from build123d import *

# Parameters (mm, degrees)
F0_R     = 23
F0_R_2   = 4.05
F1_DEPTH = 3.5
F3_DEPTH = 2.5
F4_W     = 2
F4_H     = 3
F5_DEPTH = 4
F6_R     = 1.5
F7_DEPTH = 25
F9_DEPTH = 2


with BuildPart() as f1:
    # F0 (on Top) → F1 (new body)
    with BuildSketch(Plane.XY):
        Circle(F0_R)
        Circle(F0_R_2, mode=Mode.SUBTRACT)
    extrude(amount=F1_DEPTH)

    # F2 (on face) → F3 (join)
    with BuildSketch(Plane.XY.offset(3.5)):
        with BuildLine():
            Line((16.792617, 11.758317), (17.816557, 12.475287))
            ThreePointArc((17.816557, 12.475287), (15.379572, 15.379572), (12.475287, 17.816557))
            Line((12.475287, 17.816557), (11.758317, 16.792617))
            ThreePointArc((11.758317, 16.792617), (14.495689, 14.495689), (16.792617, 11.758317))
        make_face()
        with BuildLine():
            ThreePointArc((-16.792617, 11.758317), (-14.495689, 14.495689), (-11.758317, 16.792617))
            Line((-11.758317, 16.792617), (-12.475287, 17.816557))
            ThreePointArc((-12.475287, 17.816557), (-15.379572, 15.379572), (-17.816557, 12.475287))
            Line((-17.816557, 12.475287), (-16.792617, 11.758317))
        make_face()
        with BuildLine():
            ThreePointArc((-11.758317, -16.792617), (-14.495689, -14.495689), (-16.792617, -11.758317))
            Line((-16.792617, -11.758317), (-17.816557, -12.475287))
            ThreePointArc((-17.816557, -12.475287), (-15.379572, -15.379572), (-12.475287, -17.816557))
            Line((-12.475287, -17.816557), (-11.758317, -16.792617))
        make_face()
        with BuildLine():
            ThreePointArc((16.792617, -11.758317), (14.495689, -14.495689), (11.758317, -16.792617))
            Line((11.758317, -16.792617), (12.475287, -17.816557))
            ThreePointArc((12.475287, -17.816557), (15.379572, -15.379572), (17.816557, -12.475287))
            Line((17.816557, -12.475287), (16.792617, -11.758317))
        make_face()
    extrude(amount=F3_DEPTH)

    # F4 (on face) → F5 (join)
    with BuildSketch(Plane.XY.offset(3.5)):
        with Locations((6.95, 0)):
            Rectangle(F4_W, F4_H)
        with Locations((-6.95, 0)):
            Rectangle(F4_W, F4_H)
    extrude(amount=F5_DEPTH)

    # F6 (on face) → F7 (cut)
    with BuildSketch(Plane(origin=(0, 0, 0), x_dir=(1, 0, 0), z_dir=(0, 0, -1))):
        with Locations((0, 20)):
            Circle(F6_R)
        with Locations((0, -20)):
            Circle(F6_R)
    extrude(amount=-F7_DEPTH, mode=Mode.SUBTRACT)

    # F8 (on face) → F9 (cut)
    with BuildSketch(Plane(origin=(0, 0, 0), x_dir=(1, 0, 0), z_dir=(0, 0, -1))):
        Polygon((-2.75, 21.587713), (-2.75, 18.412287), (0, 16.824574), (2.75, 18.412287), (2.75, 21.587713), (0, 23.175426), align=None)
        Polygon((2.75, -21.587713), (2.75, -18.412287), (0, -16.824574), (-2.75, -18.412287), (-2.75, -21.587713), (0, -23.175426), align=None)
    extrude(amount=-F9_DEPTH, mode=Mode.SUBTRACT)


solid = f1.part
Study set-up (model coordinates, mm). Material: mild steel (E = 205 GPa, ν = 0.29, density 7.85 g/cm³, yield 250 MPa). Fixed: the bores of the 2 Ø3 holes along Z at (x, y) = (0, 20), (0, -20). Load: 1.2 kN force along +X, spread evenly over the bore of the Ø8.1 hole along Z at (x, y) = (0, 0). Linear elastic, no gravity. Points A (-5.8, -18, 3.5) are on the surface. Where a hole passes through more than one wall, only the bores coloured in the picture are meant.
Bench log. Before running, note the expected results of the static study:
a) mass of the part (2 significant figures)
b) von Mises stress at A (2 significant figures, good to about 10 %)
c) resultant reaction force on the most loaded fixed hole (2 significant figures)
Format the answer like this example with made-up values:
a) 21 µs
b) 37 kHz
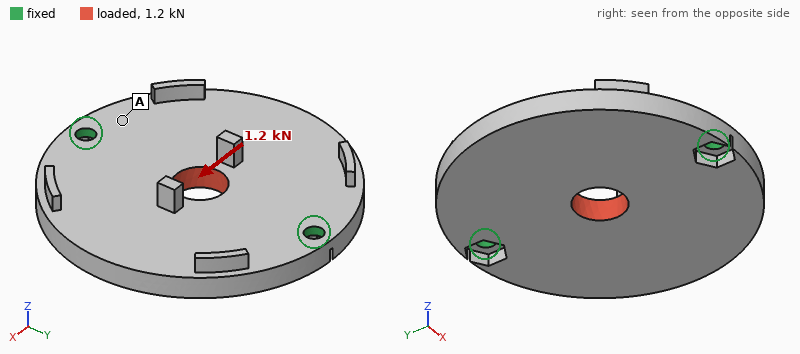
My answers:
a) 44 g
b) 18 MPa
c) 600 N
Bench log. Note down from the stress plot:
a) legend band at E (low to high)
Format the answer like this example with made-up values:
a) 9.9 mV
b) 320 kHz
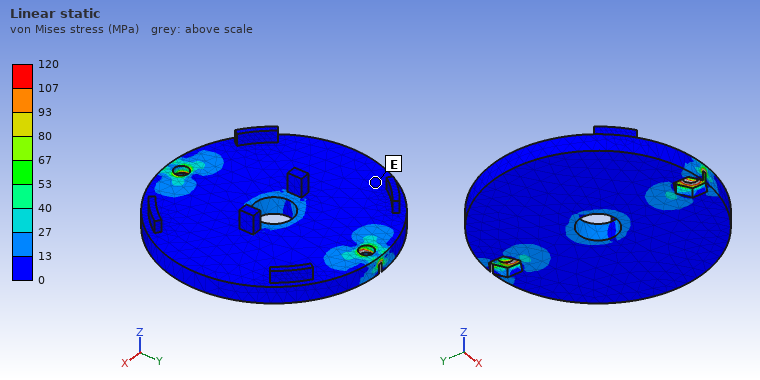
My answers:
a) 0 to 13 MPa
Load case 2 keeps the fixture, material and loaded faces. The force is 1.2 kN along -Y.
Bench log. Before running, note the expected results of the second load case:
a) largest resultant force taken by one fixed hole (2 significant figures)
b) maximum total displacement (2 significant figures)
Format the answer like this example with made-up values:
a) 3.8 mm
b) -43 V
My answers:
a) 600 N
b) 2.0 µm
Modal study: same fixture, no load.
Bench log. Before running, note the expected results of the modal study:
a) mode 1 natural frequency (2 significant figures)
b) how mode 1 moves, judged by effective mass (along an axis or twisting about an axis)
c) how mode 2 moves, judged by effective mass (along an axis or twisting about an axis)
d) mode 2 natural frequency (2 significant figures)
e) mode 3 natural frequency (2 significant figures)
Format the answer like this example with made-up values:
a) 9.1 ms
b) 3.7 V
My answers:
a) 2400 Hz
b) twisting about Y
c) along Z
d) 4700 Hz
e) 9800 Hz
